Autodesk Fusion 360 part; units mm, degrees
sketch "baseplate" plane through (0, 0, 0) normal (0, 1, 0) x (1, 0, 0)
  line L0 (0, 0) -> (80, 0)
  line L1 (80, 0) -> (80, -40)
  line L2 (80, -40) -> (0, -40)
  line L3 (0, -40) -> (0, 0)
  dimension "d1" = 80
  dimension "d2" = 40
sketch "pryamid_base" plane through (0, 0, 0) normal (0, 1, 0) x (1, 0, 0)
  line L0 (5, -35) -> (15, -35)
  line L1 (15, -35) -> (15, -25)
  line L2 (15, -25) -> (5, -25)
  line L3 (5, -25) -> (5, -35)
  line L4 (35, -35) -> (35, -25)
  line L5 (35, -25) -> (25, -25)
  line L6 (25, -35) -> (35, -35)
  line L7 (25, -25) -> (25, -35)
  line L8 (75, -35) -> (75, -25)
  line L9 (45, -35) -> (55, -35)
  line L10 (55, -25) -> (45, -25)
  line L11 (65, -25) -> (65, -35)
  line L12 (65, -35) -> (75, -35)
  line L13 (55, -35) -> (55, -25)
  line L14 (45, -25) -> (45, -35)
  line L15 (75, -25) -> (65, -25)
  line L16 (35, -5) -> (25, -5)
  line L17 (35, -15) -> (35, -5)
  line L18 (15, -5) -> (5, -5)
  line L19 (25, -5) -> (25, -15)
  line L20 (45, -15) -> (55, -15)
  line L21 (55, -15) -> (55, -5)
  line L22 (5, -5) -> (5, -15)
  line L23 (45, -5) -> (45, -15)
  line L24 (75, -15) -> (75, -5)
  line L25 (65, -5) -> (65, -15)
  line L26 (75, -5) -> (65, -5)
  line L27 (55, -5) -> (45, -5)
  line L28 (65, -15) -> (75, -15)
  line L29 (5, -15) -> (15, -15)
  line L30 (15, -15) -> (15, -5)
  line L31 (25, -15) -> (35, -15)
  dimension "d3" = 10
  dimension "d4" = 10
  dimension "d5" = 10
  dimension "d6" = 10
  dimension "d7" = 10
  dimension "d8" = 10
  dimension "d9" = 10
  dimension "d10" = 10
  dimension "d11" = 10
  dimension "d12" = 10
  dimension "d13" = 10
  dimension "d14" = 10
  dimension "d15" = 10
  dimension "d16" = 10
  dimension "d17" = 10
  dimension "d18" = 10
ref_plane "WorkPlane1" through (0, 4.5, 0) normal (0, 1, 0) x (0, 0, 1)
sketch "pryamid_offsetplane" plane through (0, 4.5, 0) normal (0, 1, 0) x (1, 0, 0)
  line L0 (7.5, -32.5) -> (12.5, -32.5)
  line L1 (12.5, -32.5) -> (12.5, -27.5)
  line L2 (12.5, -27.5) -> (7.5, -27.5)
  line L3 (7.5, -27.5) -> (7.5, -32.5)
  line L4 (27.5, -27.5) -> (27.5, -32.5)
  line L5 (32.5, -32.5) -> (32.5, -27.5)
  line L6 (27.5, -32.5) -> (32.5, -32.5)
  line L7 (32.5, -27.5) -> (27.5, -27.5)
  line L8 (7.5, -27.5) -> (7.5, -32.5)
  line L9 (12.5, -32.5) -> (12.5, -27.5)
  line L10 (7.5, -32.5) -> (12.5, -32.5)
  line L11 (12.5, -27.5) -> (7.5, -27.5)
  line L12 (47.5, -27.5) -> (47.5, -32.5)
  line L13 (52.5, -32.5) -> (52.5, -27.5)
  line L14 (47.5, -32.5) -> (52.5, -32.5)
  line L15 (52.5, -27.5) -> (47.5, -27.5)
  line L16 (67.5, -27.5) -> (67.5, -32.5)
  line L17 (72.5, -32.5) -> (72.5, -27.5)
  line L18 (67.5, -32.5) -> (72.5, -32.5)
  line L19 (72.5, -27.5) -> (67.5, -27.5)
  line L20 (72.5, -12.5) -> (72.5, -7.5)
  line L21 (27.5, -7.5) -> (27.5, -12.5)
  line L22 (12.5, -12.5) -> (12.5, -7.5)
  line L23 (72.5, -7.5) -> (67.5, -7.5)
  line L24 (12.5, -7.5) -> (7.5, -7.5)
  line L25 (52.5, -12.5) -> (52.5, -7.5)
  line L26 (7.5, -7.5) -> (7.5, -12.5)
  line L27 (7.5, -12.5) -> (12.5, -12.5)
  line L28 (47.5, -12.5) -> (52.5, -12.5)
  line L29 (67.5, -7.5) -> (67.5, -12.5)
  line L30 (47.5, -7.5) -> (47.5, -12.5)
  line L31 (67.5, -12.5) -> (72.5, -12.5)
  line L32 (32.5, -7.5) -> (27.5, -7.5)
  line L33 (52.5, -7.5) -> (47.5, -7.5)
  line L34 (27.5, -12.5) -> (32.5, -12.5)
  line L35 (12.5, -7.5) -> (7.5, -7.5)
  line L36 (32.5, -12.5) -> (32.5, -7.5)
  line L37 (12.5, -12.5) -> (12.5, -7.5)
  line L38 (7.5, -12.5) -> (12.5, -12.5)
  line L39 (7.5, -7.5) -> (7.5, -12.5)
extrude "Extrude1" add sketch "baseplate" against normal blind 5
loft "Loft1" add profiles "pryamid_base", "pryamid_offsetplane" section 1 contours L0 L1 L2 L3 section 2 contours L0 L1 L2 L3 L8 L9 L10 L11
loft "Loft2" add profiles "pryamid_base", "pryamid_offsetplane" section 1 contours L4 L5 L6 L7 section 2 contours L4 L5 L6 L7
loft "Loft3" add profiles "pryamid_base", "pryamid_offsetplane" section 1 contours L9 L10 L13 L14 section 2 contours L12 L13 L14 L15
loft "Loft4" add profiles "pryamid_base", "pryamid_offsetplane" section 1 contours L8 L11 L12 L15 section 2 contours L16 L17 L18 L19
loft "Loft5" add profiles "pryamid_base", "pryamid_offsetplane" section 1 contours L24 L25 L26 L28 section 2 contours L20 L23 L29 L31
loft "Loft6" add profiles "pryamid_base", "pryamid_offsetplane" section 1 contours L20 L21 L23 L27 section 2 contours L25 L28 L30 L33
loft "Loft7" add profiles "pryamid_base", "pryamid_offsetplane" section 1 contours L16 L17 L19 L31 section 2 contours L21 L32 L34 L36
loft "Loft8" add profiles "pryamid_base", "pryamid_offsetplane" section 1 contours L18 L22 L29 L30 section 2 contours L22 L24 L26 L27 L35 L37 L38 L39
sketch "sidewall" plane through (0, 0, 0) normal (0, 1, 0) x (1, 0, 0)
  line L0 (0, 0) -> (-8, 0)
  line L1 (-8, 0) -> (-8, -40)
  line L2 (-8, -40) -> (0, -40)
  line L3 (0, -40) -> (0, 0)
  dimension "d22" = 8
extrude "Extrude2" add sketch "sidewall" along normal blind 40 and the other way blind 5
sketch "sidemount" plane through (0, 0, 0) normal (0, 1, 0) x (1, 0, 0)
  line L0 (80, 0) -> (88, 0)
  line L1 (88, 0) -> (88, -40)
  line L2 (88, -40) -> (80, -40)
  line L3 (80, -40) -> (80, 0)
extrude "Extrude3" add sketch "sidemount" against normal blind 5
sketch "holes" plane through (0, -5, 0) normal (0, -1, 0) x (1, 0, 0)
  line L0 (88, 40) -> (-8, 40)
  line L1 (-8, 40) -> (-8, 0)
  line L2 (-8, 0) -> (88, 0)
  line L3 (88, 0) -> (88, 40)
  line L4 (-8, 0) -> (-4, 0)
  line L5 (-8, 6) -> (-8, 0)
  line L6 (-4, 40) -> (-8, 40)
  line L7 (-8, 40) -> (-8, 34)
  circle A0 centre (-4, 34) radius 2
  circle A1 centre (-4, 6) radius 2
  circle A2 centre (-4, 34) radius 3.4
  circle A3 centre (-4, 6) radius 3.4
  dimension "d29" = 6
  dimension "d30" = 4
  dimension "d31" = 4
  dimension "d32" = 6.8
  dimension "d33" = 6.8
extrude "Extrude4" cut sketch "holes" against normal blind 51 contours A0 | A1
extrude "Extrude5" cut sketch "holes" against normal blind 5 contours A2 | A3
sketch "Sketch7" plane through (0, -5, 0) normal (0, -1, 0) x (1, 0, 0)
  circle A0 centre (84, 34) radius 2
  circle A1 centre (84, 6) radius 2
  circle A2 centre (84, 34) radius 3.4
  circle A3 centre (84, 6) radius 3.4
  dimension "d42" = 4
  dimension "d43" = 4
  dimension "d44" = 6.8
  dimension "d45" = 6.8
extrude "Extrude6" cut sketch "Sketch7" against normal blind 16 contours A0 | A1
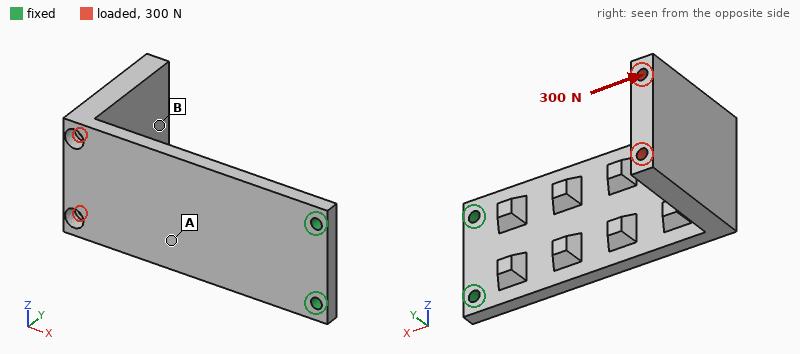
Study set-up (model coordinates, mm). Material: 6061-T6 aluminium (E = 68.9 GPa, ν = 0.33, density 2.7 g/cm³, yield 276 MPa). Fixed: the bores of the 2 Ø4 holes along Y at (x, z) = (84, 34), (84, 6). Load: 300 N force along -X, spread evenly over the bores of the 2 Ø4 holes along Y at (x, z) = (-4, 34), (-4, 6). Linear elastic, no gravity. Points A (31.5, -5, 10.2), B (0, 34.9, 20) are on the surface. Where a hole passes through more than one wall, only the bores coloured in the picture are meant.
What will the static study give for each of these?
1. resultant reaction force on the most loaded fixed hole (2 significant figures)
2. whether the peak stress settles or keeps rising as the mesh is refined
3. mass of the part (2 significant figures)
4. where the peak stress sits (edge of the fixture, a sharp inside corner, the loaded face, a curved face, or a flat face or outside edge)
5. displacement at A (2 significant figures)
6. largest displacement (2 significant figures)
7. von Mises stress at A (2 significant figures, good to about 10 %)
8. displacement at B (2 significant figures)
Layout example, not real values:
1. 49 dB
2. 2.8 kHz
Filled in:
1. 150 N
2. keeps rising
3. 88 g
4. edge of the fixture
5. 0.30 mm
6. 1.1 mm
7. 27 MPa
8. 0.98 mm
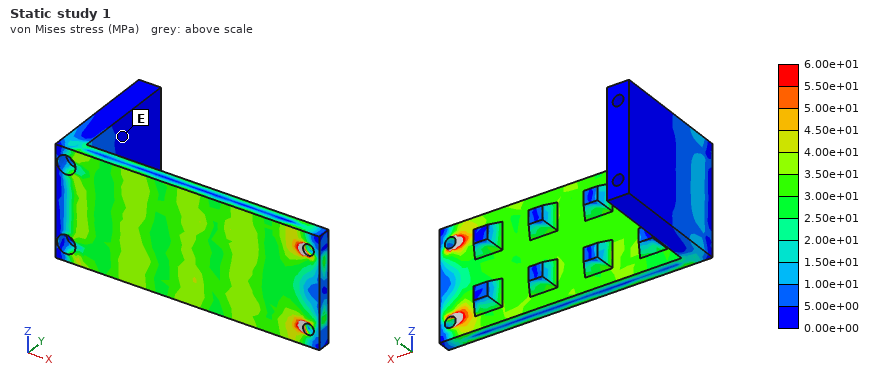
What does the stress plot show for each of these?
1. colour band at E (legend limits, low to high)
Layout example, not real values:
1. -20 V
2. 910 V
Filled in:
1. 0.00e+00 to 5.00e+00 MPa
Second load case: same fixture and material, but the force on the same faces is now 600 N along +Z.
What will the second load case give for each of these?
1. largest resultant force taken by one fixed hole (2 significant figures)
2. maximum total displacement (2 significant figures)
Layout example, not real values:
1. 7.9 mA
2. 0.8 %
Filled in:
1. 1.9 kN
2. 0.93 mm
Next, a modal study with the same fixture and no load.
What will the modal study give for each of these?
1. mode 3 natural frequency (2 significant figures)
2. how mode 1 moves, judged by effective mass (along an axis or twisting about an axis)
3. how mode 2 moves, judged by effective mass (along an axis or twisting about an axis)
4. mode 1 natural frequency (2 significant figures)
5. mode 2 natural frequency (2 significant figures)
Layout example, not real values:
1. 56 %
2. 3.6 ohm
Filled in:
1. 1200 Hz
2. along Y
3. along Z
4. 260 Hz
5. 800 Hz
